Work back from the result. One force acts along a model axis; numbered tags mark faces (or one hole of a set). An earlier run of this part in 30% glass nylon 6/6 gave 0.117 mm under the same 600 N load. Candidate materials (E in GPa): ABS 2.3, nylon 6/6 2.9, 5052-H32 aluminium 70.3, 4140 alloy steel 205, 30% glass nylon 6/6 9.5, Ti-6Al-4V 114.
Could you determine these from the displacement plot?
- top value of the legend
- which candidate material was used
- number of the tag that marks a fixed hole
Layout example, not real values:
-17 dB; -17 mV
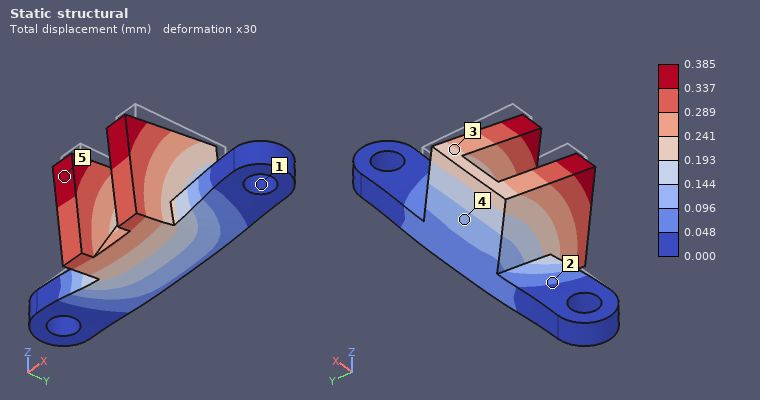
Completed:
0.385 mm; nylon 6/6; 1
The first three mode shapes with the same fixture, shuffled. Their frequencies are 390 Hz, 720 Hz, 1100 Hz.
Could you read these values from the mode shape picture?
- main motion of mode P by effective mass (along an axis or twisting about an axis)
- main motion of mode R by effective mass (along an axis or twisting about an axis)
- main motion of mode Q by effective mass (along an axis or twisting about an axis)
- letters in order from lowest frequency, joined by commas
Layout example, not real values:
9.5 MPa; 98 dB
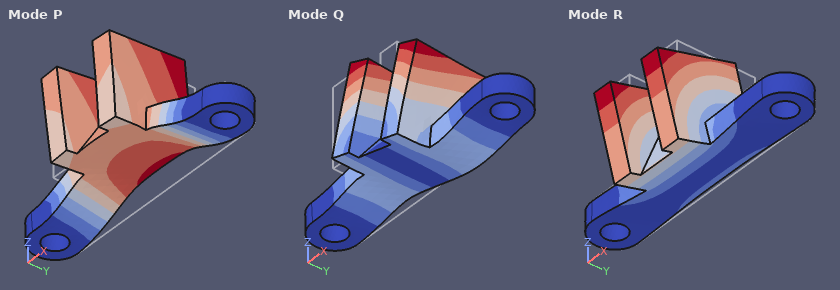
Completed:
along Z; along Y; along X; R, P, Q
